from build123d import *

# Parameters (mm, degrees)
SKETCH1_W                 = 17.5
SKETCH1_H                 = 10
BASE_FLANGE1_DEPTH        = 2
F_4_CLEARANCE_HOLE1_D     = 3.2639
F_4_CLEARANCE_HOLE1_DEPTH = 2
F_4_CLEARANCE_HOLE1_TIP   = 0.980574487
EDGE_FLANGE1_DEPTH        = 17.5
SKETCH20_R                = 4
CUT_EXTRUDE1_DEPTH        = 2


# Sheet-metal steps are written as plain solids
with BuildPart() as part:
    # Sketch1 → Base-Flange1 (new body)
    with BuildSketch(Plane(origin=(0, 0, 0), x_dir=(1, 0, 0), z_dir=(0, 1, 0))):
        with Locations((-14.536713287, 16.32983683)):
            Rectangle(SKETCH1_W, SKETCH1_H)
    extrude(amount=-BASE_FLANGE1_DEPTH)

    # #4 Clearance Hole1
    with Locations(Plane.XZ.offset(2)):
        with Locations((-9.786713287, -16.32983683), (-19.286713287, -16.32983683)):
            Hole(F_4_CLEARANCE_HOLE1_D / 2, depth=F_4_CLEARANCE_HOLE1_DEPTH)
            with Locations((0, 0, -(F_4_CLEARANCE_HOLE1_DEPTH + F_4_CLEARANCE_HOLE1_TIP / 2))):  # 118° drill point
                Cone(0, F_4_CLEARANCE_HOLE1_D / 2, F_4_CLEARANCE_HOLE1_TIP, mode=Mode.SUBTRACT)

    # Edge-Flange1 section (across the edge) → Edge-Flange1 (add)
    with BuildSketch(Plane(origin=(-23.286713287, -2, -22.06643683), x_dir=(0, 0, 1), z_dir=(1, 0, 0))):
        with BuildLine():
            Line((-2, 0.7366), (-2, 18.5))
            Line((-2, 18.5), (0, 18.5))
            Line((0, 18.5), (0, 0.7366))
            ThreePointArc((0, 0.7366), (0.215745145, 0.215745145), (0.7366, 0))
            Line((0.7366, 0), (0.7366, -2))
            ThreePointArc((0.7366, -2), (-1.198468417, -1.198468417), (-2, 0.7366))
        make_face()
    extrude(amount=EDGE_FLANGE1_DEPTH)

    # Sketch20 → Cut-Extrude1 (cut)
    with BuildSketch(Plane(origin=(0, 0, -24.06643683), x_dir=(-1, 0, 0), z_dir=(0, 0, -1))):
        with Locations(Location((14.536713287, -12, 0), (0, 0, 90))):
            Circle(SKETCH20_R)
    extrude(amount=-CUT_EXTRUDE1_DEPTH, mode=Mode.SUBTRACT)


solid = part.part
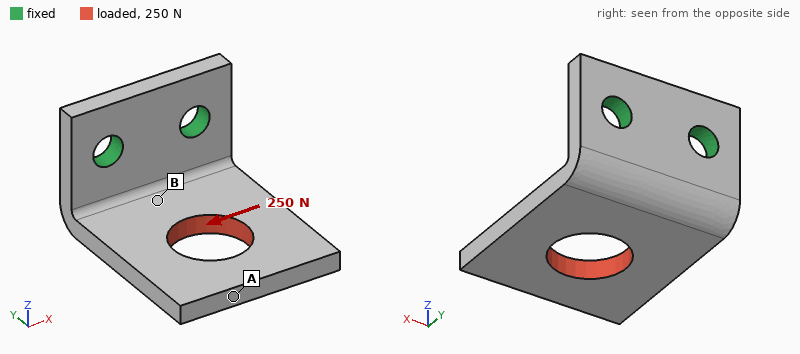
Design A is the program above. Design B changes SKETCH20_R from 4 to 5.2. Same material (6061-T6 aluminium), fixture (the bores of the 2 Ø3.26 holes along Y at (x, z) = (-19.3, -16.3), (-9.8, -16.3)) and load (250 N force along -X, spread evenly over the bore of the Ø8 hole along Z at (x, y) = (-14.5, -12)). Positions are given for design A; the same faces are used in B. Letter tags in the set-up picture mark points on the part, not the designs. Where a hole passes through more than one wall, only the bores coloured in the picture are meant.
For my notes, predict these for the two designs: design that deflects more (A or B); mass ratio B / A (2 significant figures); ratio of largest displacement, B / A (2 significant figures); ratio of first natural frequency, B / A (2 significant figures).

B
0.93
1.1
1.0
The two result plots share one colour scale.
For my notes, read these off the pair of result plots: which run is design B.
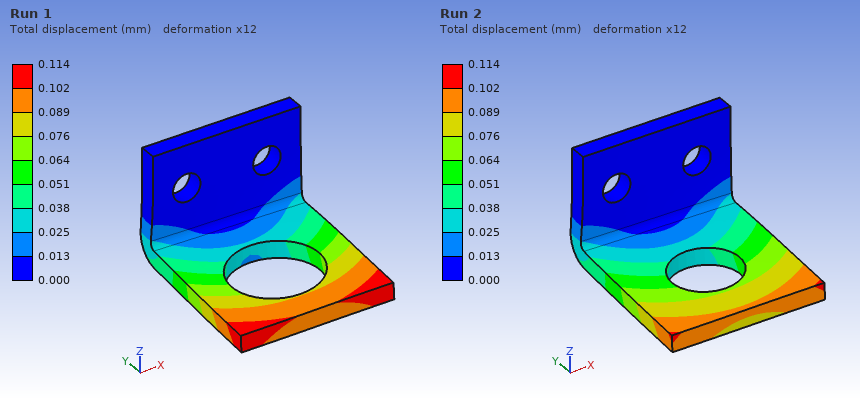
Run 1
